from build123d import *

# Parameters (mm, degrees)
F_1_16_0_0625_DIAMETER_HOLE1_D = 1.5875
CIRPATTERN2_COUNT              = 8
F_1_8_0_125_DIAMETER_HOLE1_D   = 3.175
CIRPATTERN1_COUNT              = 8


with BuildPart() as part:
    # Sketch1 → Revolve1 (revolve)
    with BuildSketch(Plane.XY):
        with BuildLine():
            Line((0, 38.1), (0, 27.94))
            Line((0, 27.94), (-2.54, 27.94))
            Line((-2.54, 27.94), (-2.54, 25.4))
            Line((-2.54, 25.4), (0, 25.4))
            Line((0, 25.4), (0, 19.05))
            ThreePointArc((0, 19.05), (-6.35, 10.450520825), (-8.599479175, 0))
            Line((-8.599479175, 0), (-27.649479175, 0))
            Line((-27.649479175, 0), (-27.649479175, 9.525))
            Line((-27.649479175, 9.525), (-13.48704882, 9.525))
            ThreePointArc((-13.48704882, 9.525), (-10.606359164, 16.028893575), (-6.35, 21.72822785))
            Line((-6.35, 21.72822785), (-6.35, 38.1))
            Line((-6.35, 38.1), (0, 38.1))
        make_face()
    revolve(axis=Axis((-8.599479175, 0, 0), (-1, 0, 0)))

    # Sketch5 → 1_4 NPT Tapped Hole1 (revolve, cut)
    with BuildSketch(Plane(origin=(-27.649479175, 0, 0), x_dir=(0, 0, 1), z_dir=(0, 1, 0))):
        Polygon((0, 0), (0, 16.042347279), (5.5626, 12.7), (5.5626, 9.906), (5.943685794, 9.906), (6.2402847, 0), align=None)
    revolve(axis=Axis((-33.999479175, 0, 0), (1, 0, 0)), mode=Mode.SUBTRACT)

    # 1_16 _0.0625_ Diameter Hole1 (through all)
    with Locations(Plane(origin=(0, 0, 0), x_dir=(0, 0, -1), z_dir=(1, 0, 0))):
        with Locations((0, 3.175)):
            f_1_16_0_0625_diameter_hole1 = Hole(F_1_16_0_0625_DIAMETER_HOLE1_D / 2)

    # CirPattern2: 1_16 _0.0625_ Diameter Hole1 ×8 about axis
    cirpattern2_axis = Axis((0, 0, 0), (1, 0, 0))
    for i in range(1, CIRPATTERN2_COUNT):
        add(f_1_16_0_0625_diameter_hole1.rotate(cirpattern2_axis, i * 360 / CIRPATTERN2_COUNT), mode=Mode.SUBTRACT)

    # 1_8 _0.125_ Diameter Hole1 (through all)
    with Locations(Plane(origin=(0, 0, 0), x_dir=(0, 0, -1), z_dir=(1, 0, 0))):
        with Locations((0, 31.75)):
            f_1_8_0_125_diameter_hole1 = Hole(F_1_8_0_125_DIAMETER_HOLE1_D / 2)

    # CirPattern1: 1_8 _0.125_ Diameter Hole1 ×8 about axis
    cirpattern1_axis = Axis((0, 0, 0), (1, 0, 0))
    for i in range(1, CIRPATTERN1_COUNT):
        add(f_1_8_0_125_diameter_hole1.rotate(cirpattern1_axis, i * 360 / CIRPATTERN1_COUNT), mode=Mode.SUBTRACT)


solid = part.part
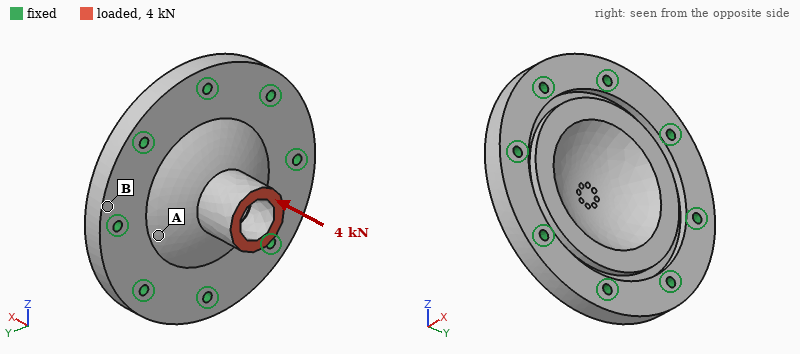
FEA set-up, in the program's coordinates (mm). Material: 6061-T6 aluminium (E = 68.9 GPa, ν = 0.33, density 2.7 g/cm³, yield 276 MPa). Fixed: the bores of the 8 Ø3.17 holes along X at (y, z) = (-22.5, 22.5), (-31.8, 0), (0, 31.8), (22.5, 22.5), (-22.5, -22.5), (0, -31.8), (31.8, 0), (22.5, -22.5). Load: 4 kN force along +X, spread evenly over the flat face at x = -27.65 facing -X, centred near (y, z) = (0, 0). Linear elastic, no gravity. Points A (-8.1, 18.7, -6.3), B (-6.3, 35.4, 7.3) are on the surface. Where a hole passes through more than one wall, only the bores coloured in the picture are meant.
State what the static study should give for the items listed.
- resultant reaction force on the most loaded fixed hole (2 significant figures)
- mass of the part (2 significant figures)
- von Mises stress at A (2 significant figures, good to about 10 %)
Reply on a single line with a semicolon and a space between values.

810 N; 84 g; 20 MPa
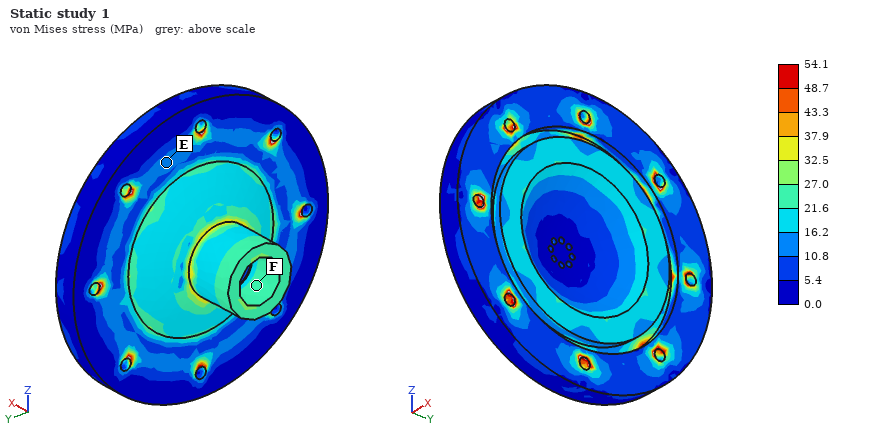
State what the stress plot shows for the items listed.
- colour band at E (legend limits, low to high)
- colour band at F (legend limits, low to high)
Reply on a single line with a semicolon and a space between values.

10.8 to 16.2 MPa; 21.6 to 27.0 MPa
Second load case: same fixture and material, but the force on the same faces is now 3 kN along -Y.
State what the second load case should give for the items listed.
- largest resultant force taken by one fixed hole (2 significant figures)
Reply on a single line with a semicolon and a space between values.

980 N
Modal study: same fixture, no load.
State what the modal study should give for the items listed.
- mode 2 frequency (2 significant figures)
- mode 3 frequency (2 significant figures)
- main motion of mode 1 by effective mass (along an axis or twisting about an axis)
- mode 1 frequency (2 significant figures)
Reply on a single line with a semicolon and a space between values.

17 kHz; 17 kHz; along X; 13 kHz
